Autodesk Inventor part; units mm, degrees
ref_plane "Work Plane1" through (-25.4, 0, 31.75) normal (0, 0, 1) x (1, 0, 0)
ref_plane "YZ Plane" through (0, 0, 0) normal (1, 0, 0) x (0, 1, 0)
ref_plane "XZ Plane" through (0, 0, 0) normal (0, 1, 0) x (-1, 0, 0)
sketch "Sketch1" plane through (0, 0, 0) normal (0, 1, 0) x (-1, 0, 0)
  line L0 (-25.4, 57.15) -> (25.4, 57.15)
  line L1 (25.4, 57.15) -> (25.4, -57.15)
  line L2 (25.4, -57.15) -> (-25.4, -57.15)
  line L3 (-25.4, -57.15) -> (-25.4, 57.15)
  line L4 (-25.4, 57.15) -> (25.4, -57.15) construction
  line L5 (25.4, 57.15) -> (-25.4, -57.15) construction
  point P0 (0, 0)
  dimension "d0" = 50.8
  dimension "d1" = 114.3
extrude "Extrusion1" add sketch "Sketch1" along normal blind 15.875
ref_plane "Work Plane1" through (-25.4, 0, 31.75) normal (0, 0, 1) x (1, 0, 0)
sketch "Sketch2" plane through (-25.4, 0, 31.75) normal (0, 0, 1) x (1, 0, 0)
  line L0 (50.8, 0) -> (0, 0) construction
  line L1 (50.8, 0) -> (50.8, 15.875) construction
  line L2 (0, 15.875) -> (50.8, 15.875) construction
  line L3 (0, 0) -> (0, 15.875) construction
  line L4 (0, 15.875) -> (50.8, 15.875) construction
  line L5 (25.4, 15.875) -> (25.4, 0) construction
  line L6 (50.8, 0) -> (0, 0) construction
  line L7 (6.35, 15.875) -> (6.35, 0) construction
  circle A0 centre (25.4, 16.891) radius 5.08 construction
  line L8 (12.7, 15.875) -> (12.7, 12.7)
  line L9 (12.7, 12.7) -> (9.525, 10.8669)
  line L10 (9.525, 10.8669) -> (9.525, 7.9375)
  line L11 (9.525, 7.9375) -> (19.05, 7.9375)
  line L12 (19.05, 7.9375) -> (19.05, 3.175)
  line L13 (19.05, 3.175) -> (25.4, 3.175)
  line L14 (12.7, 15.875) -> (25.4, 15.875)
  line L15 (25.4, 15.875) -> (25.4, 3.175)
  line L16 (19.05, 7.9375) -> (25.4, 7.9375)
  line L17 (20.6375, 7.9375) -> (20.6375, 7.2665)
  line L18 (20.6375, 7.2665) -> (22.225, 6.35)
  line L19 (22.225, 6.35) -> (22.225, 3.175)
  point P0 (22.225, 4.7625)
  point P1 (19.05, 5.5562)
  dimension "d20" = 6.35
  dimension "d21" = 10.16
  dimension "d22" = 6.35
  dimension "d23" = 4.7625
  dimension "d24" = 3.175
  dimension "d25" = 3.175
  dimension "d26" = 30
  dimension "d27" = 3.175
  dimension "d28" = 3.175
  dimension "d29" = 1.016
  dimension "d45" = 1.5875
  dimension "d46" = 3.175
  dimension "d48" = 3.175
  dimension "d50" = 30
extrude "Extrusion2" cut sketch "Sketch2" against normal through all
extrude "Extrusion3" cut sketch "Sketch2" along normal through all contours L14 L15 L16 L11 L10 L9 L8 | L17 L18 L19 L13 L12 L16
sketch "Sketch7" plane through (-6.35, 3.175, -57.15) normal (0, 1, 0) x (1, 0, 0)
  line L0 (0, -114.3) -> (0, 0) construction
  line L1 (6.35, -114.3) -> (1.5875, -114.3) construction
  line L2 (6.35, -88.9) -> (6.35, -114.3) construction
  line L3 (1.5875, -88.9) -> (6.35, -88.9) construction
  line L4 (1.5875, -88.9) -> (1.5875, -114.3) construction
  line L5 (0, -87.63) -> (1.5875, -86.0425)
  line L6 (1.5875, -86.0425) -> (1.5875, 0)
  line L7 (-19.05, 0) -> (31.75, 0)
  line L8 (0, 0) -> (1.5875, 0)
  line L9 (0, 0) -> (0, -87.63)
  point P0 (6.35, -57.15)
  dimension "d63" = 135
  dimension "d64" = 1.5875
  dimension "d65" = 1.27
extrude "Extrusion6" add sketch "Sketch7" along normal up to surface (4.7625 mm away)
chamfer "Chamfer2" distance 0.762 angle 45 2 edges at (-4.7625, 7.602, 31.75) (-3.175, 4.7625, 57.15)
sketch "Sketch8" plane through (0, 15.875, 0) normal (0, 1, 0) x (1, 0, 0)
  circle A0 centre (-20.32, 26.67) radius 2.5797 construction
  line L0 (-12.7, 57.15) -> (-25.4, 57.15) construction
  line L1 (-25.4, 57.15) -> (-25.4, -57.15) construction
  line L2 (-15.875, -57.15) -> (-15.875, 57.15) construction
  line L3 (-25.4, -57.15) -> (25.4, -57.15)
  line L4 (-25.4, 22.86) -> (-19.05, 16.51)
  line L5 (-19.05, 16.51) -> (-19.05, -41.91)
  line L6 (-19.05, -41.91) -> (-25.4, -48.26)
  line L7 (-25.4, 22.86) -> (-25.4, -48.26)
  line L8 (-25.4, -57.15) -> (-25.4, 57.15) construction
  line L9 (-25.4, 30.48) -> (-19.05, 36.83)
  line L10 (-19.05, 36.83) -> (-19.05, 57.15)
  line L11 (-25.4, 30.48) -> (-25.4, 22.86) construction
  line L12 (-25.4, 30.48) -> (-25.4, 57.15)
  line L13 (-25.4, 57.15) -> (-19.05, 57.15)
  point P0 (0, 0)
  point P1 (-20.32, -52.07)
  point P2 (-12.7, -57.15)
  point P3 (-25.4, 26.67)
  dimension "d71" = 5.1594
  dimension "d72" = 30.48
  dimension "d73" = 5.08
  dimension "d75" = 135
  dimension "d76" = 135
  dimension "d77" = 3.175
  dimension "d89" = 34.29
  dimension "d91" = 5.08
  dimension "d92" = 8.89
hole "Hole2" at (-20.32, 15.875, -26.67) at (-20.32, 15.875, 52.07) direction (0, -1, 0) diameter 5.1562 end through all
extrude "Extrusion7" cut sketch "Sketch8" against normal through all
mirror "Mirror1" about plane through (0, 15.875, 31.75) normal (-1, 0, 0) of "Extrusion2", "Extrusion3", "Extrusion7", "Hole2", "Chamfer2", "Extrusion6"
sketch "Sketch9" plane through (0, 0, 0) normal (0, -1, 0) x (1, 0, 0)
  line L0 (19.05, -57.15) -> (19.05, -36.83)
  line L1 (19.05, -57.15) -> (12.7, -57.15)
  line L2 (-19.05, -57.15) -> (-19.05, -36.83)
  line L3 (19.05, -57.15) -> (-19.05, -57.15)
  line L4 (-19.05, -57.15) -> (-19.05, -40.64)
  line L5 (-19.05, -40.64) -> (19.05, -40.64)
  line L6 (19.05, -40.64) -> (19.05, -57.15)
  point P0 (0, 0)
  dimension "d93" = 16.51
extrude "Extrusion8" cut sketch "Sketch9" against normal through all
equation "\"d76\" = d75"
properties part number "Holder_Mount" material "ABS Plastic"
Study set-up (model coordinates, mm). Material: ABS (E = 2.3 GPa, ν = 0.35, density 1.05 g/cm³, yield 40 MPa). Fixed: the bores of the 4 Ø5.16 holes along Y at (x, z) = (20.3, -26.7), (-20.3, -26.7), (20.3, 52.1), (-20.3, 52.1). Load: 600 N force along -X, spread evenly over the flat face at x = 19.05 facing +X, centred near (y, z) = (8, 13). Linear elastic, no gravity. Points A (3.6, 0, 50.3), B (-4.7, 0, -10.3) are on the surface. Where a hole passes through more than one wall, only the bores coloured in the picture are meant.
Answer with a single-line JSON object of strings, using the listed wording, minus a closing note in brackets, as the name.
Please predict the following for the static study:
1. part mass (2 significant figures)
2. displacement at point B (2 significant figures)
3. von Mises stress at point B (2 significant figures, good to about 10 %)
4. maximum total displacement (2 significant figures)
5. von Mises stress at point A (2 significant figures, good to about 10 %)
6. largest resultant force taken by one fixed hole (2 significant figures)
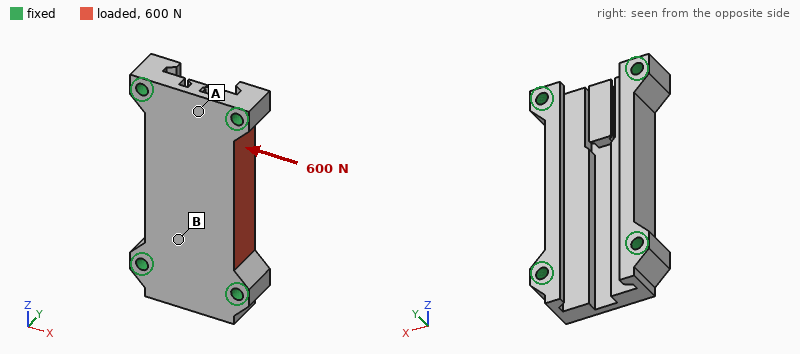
{"part mass": "39 g", "displacement at point B": "0.047 mm", "von Mises stress at point B": "3.0 MPa", "maximum total displacement": "0.26 mm", "von Mises stress at point A": "1.2 MPa", "largest resultant force taken by one fixed hole": "270 N"}
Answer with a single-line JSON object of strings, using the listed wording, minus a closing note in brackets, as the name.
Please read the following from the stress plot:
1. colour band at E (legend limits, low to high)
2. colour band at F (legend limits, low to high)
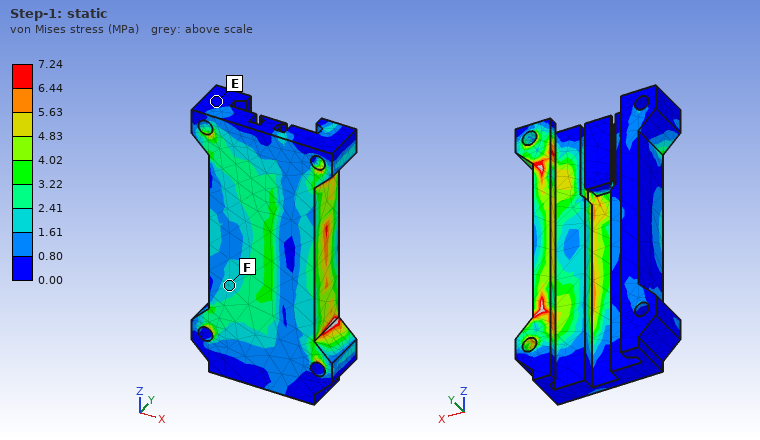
{"colour band at E": "0.00 to 0.80 MPa", "colour band at F": "1.61 to 2.41 MPa"}
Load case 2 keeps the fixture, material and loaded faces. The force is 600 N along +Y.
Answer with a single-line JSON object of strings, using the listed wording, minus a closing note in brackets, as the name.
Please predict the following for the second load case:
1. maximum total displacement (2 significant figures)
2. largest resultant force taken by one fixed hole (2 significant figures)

{"maximum total displacement": "0.33 mm", "largest resultant force taken by one fixed hole": "300 N"}
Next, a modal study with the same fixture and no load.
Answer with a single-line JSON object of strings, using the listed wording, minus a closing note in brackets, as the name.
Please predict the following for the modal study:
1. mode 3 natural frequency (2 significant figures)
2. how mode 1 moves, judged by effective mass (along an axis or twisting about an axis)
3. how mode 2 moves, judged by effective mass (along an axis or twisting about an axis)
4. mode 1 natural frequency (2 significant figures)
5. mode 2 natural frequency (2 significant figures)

{"mode 3 natural frequency": "3800 Hz", "how mode 1 moves, judged by effective mass": "along Y", "how mode 2 moves, judged by effective mass": "along X", "mode 1 natural frequency": "2500 Hz", "mode 2 natural frequency": "3200 Hz"}
